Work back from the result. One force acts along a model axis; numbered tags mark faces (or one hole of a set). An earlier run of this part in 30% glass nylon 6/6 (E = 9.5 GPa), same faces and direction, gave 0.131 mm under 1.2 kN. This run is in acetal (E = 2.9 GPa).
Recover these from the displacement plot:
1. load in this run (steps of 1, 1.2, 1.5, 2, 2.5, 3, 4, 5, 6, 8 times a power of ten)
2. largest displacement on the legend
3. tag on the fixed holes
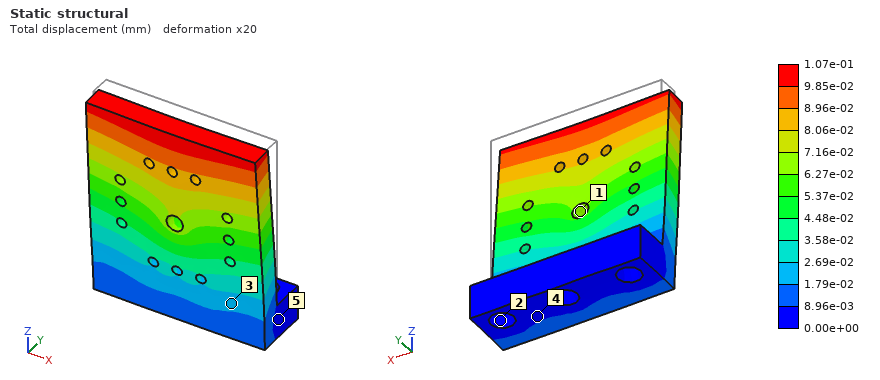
300 N
1.07e-01 mm
2
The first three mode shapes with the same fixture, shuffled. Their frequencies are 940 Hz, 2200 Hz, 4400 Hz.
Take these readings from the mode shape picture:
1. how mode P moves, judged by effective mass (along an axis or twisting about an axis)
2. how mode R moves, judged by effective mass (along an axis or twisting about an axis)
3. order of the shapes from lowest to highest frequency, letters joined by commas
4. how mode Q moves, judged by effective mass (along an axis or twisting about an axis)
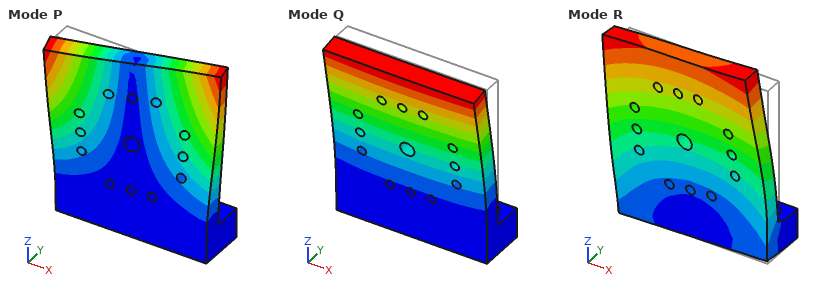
twisting about Z
along X
Q, P, R
along Y
